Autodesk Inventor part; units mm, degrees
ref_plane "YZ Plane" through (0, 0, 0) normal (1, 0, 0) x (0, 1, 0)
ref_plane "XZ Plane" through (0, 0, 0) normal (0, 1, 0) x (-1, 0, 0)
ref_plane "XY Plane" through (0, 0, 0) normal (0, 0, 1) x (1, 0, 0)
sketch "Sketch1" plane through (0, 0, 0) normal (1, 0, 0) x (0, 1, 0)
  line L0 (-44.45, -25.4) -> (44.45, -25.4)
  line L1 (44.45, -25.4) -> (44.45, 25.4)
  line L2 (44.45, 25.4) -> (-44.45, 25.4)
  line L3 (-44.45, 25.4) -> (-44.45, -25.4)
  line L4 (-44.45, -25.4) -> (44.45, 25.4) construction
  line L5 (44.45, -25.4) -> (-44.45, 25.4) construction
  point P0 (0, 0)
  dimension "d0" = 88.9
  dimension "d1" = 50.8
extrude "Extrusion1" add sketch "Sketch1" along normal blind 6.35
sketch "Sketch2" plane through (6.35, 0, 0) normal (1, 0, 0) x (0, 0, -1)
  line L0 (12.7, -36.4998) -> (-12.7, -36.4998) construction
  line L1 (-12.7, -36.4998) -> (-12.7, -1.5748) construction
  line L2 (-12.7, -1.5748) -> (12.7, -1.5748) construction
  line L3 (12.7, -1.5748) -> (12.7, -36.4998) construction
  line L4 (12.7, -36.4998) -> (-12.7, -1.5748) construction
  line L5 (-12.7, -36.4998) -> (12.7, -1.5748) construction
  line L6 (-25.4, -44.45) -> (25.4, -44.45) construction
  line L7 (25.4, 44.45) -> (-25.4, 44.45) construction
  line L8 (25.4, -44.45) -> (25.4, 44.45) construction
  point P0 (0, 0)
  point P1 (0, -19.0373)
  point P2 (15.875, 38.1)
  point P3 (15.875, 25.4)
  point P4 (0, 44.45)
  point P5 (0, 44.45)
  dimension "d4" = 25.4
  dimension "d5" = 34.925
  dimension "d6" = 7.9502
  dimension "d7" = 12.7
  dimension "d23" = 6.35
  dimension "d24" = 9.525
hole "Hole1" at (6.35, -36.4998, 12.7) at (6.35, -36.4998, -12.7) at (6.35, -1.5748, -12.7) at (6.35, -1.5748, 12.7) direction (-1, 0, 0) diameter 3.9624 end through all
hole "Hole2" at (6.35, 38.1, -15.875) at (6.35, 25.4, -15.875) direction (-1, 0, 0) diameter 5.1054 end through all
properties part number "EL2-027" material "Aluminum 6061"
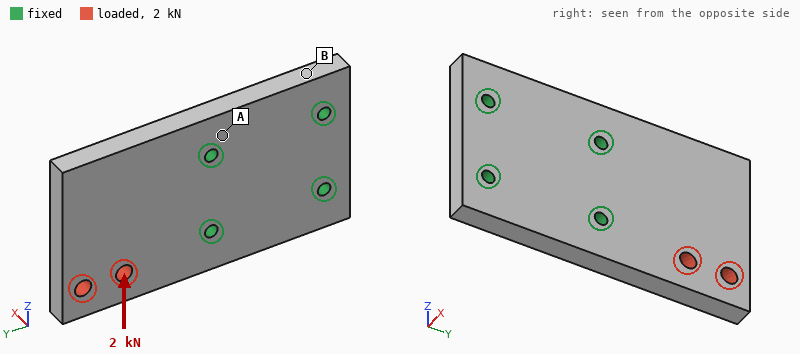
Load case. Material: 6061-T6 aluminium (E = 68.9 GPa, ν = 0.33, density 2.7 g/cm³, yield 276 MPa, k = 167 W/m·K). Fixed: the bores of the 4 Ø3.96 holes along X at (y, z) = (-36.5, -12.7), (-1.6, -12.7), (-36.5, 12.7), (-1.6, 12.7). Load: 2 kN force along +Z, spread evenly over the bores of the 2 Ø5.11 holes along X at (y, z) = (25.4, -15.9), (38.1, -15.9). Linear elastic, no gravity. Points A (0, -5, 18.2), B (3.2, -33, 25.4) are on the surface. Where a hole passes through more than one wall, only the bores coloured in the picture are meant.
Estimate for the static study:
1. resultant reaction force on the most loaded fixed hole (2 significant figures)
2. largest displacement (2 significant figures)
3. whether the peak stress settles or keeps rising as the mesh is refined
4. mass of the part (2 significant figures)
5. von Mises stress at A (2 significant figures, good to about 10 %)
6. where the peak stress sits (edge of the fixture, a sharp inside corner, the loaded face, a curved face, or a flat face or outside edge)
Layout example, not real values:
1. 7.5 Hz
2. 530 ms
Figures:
1. 2.0 kN
2. 28 µm
3. keeps rising
4. 76 g
5. 12 MPa
6. edge of the fixture
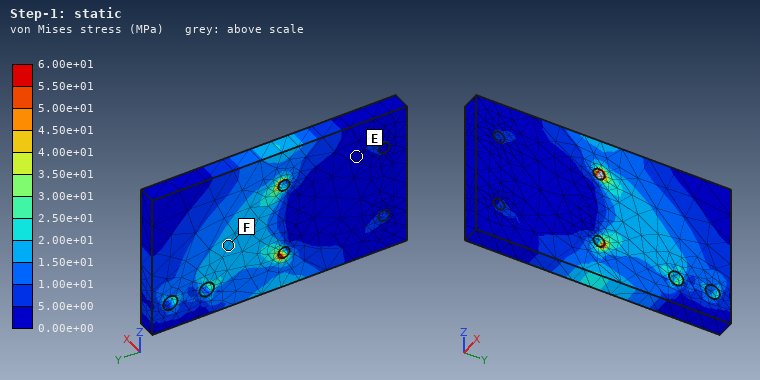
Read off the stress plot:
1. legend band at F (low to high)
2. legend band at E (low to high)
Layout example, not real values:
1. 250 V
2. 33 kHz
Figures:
1. 1.50e+01 to 2.00e+01 MPa
2. 0.00e+00 to 5.00e+00 MPa
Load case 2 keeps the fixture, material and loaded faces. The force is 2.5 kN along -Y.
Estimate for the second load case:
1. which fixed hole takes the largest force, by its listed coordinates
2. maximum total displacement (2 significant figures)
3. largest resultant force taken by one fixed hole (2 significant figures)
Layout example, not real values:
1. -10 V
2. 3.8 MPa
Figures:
1. (-1.6, -12.7)
2. 16 µm
3. 2.1 kN
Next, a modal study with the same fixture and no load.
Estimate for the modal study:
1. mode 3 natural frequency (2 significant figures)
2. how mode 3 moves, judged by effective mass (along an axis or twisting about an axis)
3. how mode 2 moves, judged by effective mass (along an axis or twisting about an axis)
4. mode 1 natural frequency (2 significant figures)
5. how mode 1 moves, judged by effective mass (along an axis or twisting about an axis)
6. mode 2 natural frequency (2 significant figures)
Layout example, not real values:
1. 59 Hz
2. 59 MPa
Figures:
1. 10 kHz
2. along Z
3. twisting about Y
4. 2400 Hz
5. along X
6. 5000 Hz
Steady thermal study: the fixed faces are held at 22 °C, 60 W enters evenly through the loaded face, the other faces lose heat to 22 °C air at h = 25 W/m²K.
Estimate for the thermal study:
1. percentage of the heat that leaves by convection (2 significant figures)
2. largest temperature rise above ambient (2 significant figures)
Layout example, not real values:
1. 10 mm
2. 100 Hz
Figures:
1. 6.1 %
2. 58 K
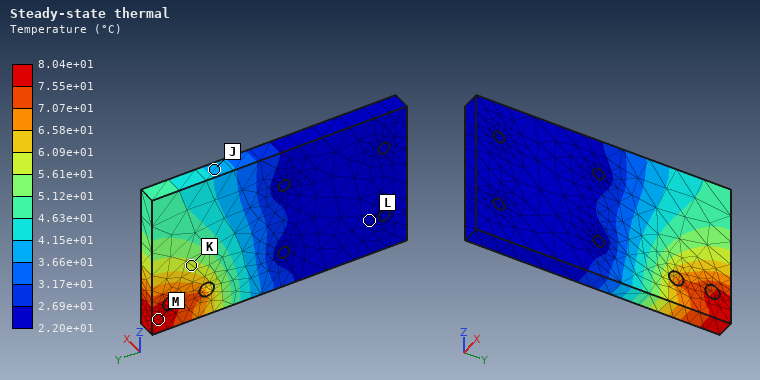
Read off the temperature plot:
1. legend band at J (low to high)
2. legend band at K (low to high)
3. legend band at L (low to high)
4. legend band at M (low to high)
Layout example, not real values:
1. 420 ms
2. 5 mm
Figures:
1. 3.66e+01 to 4.15e+01 °C
2. 5.61e+01 to 6.09e+01 °C
3. 2.20e+01 to 2.69e+01 °C
4. 7.55e+01 to 8.04e+01 °C
